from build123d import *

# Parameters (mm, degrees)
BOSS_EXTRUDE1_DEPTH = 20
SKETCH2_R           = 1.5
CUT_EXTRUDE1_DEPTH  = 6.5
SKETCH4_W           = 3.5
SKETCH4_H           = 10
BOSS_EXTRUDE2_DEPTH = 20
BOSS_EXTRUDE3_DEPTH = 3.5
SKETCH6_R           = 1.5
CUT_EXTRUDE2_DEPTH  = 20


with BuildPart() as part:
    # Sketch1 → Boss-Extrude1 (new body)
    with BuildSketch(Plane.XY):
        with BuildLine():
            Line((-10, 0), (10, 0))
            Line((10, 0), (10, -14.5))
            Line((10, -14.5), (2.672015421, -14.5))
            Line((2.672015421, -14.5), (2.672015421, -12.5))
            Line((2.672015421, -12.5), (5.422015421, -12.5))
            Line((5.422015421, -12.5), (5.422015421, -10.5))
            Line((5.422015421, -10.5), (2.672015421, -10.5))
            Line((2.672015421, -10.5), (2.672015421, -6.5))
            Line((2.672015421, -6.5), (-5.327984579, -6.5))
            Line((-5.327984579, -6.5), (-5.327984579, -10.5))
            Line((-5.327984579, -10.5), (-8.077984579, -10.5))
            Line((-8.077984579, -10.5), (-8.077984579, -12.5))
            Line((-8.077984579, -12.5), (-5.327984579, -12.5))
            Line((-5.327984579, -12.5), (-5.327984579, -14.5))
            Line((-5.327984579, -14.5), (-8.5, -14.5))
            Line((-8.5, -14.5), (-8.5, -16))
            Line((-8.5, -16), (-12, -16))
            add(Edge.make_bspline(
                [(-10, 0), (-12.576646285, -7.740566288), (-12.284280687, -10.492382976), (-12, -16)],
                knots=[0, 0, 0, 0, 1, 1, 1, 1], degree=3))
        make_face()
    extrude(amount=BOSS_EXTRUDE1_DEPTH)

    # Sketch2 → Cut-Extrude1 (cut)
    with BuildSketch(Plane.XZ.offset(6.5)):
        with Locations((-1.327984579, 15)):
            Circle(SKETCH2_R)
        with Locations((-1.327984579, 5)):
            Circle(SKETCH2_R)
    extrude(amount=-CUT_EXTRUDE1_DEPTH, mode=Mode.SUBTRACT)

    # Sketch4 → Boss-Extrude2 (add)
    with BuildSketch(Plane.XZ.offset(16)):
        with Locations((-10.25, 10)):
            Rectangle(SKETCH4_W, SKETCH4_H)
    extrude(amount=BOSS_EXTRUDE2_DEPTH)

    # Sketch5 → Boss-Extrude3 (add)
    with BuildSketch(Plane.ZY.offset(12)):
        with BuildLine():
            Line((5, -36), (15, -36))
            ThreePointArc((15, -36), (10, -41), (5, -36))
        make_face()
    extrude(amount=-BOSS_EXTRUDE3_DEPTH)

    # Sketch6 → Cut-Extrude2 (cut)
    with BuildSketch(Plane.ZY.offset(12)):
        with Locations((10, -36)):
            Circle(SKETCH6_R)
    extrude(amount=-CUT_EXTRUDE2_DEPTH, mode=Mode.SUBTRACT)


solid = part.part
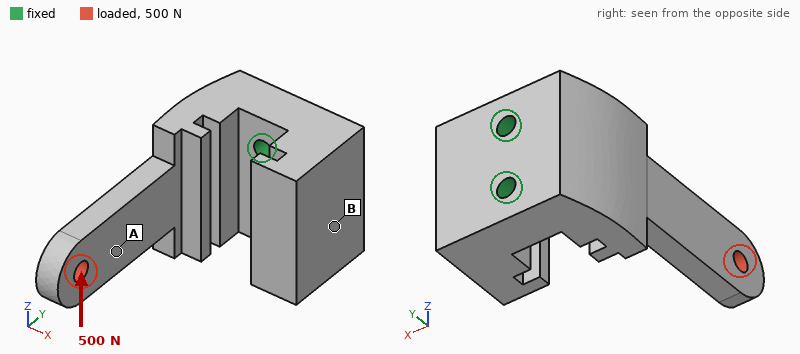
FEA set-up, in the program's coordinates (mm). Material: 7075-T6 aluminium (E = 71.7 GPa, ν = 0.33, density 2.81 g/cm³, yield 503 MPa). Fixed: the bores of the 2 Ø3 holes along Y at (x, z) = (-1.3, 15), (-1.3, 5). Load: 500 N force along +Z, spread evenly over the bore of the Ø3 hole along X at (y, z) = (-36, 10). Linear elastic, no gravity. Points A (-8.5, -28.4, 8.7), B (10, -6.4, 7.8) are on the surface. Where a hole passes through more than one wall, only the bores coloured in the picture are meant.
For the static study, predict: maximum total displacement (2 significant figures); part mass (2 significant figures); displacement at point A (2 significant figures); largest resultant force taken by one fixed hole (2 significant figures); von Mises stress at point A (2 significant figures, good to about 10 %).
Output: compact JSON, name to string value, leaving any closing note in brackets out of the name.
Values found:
{"maximum total displacement": "0.21 mm", "part mass": "16 g", "displacement at point A": "0.10 mm", "largest resultant force taken by one fixed hole": "1.2 kN", "von Mises stress at point A": "39 MPa"}
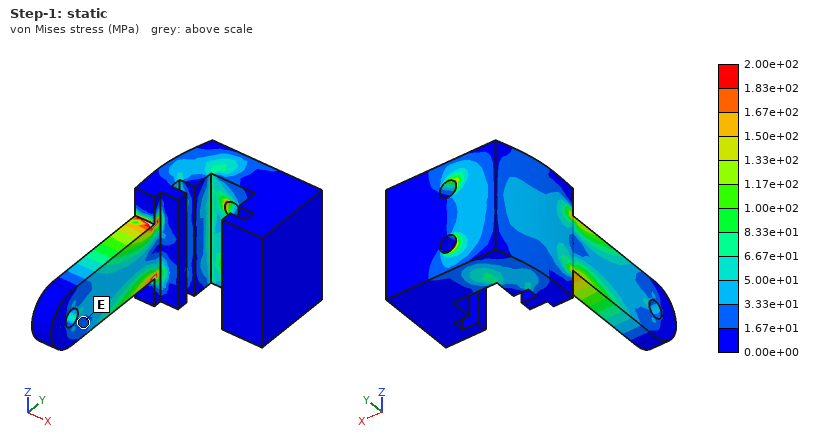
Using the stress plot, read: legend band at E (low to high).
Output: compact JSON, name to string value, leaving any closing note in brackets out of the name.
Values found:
{"legend band at E": "1.67e+01 to 3.33e+01 MPa"}
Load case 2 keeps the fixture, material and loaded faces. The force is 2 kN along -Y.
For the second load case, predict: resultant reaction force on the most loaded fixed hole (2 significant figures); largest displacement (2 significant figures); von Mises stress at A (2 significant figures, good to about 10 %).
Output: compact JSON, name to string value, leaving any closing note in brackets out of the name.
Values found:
{"resultant reaction force on the most loaded fixed hole": "1.0 kN", "largest displacement": "0.13 mm", "von Mises stress at A": "58 MPa"}
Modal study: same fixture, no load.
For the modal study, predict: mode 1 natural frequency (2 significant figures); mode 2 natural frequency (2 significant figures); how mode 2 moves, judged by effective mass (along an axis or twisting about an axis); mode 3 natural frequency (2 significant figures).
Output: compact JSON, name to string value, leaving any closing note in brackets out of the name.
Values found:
{"mode 1 natural frequency": "3400 Hz", "mode 2 natural frequency": "8200 Hz", "how mode 2 moves, judged by effective mass": "along Z", "mode 3 natural frequency": "14 kHz"}
